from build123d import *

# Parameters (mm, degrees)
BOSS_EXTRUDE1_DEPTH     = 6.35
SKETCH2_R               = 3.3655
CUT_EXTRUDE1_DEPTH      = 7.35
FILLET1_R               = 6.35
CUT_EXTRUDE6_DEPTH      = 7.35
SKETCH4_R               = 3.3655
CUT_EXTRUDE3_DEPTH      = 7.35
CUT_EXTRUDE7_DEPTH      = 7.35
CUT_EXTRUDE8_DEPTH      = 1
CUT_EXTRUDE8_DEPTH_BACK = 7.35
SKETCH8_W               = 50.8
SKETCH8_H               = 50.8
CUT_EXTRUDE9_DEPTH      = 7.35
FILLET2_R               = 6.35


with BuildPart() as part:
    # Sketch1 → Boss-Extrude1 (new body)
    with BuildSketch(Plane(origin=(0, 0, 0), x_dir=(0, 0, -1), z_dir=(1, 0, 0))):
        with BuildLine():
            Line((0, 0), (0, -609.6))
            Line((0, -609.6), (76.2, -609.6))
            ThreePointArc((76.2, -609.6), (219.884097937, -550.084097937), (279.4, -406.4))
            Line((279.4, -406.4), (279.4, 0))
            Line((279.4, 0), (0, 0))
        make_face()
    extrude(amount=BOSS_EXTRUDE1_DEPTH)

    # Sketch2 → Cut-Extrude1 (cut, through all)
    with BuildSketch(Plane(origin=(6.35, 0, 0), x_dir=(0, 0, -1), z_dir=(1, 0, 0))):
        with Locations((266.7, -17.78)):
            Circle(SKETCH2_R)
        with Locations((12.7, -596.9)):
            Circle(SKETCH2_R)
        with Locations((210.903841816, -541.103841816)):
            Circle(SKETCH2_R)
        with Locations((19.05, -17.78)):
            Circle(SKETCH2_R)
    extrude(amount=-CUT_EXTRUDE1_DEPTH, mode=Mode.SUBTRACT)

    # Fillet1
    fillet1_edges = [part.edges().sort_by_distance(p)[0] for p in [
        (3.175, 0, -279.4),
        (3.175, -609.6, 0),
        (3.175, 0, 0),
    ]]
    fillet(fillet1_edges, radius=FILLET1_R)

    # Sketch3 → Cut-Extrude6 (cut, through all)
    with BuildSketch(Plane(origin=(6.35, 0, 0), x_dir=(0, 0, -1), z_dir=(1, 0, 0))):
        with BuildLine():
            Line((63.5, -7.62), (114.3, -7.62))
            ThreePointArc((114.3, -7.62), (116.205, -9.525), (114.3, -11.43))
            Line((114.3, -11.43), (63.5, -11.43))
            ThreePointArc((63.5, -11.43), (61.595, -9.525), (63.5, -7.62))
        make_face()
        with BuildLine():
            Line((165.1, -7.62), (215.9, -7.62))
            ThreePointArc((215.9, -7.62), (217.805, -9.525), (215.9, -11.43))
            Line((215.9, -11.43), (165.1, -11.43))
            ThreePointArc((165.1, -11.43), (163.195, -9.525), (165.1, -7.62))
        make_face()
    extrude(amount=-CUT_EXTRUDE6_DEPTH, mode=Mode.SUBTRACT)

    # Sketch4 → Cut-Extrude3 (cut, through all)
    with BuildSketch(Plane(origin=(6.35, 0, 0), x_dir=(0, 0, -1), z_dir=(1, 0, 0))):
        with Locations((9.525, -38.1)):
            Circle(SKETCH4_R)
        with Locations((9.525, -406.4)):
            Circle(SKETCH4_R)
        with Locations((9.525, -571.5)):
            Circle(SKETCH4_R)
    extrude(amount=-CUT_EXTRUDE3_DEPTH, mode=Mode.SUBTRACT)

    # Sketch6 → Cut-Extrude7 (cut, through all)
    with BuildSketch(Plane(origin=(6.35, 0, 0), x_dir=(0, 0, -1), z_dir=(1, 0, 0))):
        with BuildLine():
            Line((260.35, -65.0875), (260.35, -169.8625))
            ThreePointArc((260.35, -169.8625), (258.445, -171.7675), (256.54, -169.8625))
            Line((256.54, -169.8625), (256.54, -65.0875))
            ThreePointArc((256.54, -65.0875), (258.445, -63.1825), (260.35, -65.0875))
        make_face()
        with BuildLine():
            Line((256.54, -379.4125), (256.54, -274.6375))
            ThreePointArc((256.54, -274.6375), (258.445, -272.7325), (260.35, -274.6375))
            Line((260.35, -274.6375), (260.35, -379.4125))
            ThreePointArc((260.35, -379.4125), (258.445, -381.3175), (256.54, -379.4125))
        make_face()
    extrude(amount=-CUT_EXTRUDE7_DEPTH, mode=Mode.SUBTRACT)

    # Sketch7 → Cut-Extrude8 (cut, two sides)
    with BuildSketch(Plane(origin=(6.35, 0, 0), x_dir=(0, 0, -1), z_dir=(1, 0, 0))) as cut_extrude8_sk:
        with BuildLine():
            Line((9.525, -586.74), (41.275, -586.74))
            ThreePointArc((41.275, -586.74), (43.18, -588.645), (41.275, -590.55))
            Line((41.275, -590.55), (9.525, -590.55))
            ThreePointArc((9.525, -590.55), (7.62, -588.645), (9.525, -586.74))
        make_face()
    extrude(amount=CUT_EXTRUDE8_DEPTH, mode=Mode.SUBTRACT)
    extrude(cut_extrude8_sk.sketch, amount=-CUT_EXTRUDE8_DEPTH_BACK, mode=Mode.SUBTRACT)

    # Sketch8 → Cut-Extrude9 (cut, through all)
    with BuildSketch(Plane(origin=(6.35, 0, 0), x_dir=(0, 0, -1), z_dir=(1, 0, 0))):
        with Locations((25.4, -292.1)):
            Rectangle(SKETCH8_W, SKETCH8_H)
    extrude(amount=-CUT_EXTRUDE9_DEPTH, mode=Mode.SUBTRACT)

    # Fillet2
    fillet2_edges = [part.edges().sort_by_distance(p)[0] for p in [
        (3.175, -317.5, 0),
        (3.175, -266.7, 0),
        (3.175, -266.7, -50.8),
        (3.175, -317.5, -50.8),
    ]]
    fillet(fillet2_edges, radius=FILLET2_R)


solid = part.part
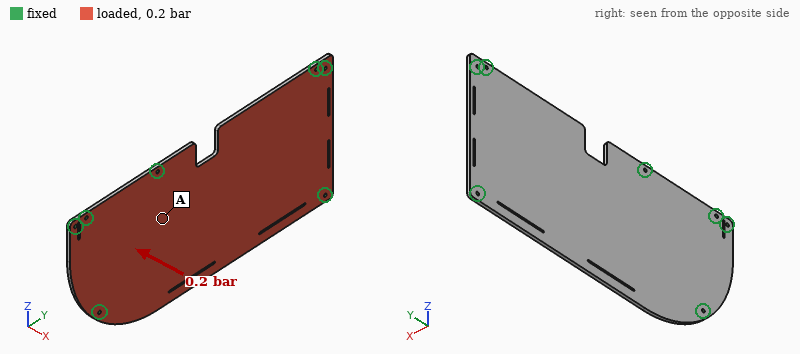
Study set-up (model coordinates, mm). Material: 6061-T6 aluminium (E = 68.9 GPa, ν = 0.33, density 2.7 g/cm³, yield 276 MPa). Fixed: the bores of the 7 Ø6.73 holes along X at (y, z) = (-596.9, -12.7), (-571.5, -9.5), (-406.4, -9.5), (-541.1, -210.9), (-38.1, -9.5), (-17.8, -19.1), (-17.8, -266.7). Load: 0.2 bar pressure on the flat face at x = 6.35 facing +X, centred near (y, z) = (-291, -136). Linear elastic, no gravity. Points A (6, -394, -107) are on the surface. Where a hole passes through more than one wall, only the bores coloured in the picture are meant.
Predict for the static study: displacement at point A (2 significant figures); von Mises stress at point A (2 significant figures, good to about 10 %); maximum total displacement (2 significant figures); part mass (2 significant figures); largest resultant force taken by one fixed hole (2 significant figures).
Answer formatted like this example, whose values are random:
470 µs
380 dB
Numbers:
0.93 mm
14 MPa
3.3 mm
2.7 kg
980 N
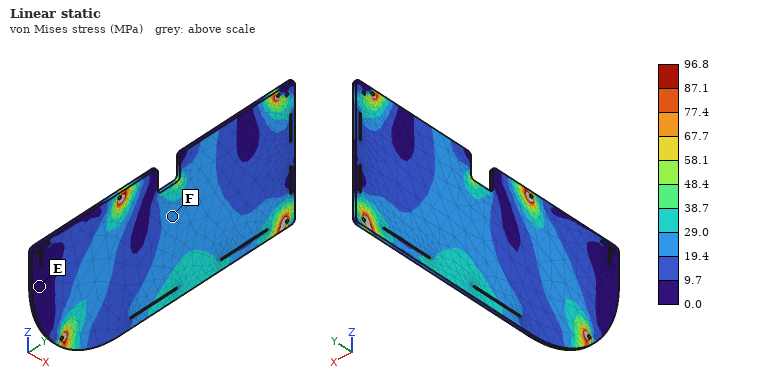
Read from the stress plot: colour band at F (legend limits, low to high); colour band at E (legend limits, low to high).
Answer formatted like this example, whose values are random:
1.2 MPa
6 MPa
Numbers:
19.4 to 29.0 MPa
0.0 to 9.7 MPa
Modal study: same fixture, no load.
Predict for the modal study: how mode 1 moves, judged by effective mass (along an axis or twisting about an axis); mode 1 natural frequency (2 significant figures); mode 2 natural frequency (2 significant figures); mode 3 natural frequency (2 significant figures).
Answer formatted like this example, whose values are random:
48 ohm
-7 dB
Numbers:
along X
120 Hz
240 Hz
330 Hz
